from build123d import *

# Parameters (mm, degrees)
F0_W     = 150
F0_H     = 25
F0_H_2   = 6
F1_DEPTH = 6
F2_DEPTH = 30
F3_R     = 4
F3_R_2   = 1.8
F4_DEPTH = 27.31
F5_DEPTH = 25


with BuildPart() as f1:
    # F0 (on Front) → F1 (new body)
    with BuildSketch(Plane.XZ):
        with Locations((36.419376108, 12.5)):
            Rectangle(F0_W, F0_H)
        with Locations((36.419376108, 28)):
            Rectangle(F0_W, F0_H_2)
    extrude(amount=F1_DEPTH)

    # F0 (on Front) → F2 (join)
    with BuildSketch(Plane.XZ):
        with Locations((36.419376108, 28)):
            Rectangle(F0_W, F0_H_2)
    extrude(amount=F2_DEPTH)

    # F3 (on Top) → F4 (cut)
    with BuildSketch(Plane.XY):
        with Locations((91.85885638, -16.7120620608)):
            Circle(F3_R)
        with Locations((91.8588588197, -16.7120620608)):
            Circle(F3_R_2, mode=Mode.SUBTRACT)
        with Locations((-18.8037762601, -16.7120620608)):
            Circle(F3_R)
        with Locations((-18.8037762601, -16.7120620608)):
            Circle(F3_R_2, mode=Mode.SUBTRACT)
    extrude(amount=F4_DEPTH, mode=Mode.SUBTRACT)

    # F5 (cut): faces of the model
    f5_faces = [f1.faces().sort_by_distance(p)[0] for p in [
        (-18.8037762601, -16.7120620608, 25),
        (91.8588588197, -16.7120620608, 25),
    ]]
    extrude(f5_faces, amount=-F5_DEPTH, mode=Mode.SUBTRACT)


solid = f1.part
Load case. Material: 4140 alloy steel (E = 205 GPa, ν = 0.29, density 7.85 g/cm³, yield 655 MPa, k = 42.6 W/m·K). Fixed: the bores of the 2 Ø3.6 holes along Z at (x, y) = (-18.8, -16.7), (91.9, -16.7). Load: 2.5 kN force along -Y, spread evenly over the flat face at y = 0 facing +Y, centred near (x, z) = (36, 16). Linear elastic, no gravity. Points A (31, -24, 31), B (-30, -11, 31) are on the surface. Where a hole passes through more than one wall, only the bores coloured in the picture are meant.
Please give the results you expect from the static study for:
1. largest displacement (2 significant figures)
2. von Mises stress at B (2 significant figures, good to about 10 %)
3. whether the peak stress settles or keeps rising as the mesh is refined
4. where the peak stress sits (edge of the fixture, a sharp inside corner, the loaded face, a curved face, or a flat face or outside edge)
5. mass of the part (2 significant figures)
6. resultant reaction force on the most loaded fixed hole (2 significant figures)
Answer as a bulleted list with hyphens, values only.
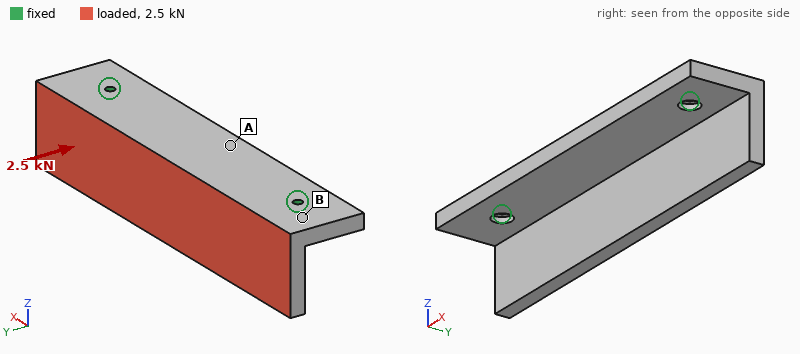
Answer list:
- 0.13 mm
- 44 MPa
- keeps rising
- edge of the fixture
- 390 g
- 1.3 kN
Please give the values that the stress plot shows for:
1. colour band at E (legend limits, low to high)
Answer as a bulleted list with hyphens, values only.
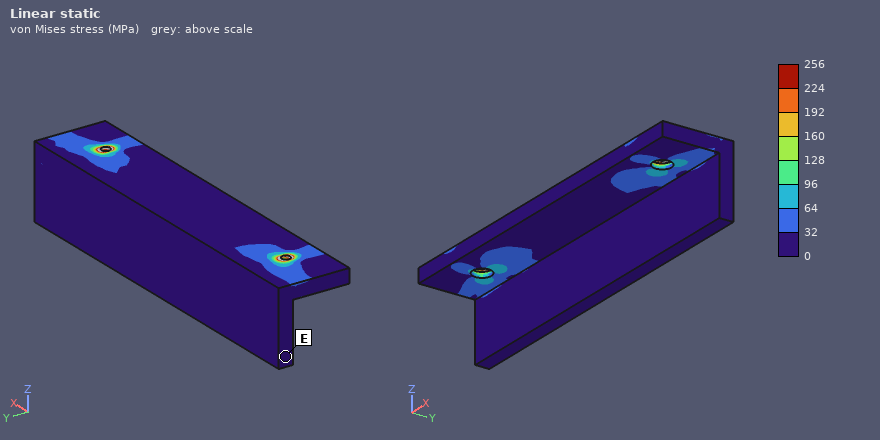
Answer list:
- 0 to 32 MPa
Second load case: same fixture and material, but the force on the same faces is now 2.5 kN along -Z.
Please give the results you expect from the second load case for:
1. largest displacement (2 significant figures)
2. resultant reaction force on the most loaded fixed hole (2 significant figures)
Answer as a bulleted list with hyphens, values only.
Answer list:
- 0.12 mm
- 1.3 kN
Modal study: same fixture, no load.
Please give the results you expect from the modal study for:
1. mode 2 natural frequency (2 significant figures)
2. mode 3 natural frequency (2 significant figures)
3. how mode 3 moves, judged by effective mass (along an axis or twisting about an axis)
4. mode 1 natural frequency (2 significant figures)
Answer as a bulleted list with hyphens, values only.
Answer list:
- 2900 Hz
- 3600 Hz
- along Z
- 1600 Hz
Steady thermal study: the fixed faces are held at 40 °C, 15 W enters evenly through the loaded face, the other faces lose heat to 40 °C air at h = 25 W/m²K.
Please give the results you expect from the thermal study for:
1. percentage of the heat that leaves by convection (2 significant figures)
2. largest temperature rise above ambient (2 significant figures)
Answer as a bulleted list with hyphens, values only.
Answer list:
- 31 %
- 20 K
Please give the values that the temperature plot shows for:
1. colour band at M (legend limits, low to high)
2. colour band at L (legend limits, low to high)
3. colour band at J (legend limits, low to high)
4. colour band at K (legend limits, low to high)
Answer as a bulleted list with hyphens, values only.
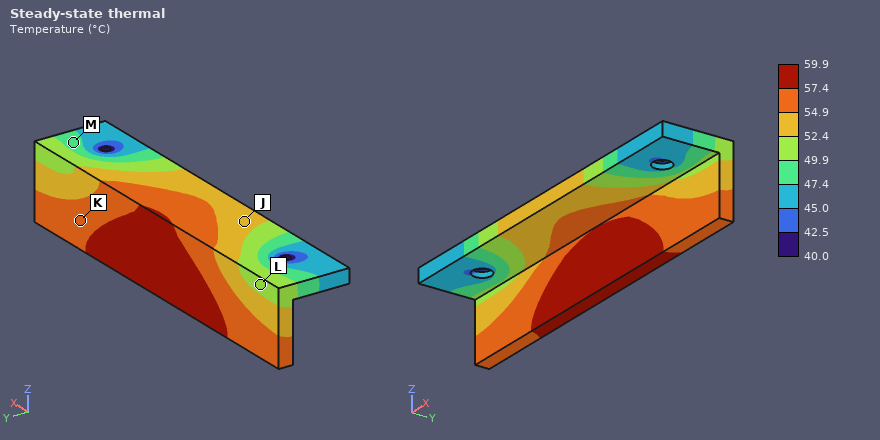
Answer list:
- 47.4 to 49.9 °C
- 49.9 to 52.4 °C
- 52.4 to 54.9 °C
- 54.9 to 57.4 °C
